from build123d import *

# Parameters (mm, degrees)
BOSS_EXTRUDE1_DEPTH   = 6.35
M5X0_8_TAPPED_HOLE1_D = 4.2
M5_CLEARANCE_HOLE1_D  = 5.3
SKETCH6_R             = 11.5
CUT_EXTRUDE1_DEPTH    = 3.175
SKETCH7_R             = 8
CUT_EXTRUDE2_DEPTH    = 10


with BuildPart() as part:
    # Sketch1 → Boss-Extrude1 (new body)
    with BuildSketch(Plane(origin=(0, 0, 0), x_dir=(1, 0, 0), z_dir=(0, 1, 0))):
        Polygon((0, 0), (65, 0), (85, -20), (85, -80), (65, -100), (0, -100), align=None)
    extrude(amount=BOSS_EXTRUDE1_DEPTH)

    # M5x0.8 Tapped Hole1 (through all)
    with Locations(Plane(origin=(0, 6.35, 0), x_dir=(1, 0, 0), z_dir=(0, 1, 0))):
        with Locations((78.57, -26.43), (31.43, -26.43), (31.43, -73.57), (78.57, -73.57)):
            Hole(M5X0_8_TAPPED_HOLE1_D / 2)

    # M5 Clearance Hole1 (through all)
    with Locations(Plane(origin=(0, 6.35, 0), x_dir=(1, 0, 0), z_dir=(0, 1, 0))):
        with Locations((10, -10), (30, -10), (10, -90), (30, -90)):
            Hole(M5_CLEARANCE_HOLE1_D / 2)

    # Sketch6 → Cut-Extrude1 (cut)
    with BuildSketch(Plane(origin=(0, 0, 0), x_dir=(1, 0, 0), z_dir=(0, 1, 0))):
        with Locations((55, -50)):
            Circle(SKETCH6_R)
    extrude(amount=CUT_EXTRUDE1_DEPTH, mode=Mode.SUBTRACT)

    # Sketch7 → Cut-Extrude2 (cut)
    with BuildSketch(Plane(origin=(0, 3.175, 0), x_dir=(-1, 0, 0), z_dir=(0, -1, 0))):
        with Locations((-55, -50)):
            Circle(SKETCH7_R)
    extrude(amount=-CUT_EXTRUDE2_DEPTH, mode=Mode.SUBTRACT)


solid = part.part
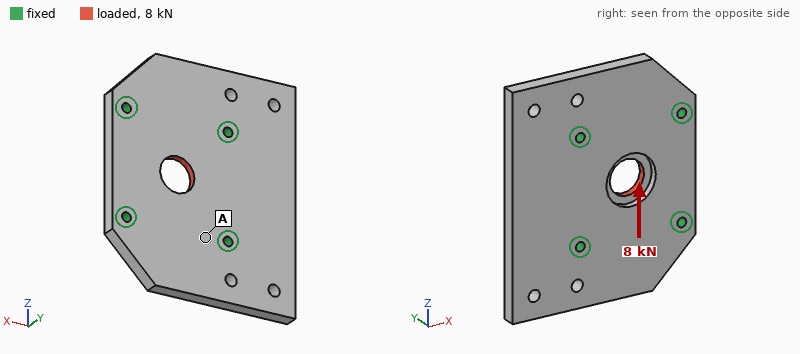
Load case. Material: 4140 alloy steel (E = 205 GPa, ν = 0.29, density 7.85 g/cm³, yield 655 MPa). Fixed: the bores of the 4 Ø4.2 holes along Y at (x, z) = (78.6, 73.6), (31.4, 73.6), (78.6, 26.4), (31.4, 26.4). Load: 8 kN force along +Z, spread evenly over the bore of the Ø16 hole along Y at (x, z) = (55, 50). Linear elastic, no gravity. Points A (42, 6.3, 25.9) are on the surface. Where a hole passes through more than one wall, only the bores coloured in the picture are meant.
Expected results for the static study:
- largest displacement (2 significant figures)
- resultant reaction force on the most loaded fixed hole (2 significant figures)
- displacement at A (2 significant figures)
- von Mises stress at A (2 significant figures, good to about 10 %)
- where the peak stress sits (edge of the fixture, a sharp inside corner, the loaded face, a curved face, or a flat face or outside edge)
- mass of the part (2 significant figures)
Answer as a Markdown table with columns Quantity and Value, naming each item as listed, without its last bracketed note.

| Quantity | Value |
|---|---|
| largest displacement | 5.0 µm |
| resultant reaction force on the most loaded fixed hole | 2.1 kN |
| displacement at A | 1.4 µm |
| von Mises stress at A | 13 MPa |
| where the peak stress sits | a sharp inside corner |
| mass of the part | 380 g |
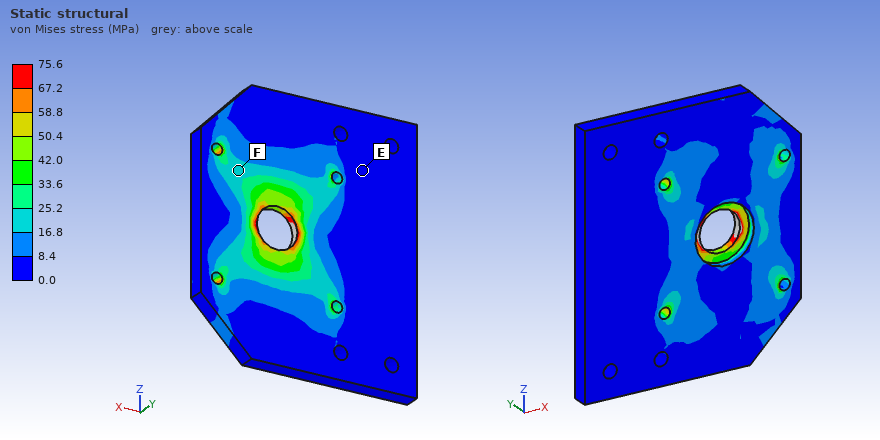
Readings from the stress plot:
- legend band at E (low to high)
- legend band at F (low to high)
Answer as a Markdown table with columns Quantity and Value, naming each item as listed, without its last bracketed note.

| Quantity | Value |
|---|---|
| legend band at E | 0.0 to 8.4 MPa |
| legend band at F | 16.8 to 25.2 MPa |
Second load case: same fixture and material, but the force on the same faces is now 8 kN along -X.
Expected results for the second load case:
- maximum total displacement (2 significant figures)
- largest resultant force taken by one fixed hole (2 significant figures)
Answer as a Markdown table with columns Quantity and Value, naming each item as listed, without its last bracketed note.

| Quantity | Value |
|---|---|
| maximum total displacement | 5.8 µm |
| largest resultant force taken by one fixed hole | 2.3 kN |
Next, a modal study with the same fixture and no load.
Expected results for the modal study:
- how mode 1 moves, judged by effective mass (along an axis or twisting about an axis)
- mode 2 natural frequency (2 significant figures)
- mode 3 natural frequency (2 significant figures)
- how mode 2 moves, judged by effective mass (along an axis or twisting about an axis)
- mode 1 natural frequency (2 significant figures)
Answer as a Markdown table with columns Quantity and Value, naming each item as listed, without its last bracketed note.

| Quantity | Value |
|---|---|
| how mode 1 moves, judged by effective mass | along Y |
| mode 2 natural frequency | 4700 Hz |
| mode 3 natural frequency | 5400 Hz |
| how mode 2 moves, judged by effective mass | twisting about X |
| mode 1 natural frequency | 4100 Hz |
